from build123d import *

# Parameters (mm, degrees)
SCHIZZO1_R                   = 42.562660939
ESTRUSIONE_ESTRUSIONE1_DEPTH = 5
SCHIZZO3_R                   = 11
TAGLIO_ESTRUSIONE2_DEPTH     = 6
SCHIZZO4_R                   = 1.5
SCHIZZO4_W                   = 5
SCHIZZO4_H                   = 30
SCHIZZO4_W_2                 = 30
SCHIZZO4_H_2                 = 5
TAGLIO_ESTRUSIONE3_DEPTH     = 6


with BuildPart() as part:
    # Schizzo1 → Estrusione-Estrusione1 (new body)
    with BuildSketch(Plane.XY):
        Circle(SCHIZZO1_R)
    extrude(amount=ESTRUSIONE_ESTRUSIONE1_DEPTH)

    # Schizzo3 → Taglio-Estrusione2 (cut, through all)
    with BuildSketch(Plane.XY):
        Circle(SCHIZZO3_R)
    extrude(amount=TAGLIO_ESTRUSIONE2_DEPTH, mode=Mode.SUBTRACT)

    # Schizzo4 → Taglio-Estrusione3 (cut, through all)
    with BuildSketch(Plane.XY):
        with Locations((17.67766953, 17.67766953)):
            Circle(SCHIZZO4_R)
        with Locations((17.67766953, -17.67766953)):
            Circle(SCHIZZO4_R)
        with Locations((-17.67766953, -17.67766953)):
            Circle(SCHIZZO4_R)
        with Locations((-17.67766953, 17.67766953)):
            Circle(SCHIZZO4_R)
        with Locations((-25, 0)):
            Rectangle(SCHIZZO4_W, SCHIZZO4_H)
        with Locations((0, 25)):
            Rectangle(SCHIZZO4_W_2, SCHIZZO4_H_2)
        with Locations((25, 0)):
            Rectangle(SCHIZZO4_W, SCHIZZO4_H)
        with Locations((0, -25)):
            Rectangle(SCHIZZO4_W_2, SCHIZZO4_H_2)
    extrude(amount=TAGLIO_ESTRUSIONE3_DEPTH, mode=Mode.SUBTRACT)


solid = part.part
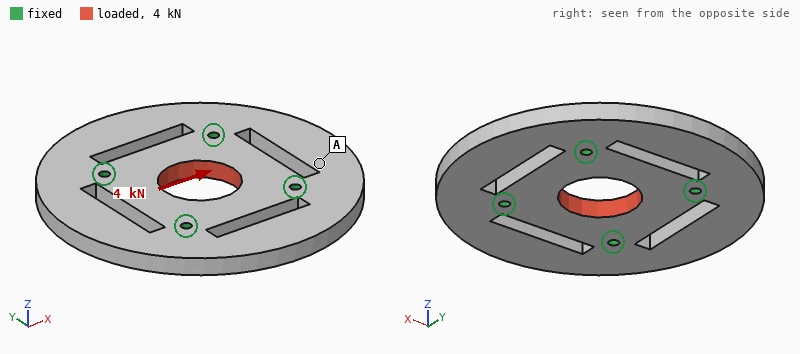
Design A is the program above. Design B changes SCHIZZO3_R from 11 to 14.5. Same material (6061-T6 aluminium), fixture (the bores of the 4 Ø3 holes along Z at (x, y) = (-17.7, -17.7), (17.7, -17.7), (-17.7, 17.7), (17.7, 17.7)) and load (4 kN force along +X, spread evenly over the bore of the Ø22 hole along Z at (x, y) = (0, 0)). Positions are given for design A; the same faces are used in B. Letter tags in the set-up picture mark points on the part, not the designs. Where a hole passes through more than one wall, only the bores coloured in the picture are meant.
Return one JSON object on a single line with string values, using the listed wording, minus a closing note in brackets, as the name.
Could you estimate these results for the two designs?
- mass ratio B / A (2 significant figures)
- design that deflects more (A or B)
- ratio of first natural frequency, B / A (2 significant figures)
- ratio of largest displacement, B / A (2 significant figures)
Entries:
{"mass ratio B / A": "0.94", "design that deflects more": "B", "ratio of first natural frequency, B / A": "1.00", "ratio of largest displacement, B / A": "1.3"}
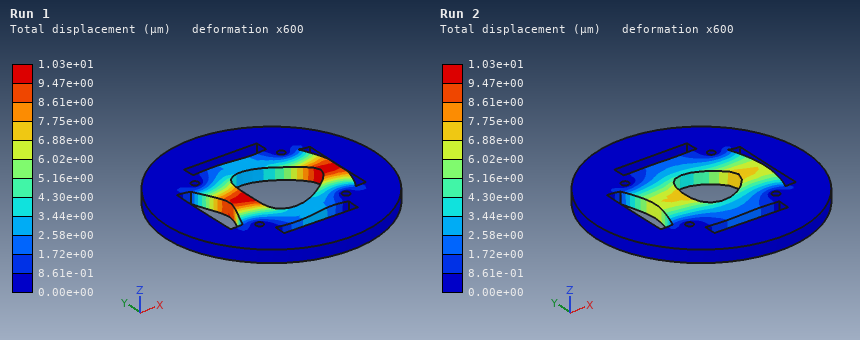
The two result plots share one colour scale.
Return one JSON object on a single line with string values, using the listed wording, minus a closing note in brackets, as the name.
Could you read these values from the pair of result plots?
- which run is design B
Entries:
{"which run is design B": "Run 1"}
